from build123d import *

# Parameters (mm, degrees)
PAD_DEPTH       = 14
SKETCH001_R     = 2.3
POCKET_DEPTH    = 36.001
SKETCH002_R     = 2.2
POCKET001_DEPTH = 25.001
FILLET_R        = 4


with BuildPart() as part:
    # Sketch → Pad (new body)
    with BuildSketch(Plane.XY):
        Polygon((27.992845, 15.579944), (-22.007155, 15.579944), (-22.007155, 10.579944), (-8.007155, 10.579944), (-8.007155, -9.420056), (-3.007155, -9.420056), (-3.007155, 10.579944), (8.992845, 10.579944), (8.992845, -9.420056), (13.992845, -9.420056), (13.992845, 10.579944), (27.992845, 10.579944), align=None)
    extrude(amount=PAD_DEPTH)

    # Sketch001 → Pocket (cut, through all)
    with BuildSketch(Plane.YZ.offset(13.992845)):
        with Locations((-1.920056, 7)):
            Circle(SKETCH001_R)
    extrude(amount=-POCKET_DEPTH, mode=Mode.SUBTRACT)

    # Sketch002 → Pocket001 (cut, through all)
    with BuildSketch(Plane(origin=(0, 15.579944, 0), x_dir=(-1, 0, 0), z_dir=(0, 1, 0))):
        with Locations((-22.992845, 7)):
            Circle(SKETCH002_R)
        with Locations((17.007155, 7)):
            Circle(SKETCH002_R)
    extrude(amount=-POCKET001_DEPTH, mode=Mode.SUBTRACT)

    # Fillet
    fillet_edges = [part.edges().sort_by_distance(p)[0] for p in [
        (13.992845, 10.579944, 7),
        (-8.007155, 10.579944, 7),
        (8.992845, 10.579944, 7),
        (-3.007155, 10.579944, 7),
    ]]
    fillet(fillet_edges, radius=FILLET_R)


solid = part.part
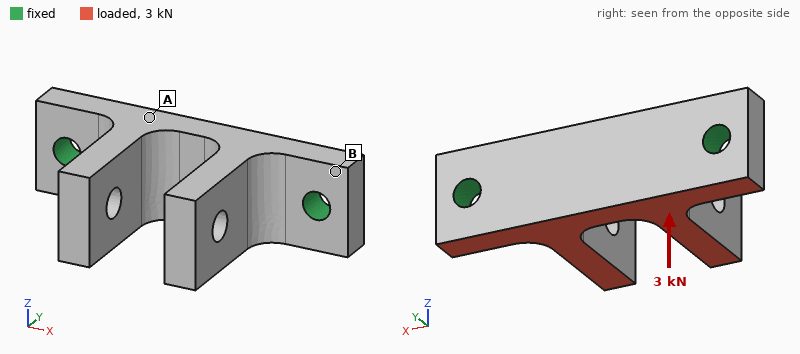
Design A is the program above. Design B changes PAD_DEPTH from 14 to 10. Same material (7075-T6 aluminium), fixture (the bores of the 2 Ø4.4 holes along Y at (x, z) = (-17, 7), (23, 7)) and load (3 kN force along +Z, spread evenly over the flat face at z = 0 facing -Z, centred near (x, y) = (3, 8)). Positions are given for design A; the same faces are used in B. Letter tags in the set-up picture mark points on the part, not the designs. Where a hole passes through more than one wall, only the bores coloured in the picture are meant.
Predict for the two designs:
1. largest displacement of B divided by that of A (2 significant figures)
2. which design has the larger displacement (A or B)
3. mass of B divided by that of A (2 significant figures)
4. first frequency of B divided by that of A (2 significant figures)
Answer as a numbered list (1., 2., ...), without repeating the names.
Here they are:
1. 1.8
2. B
3. 0.70
4. 0.93
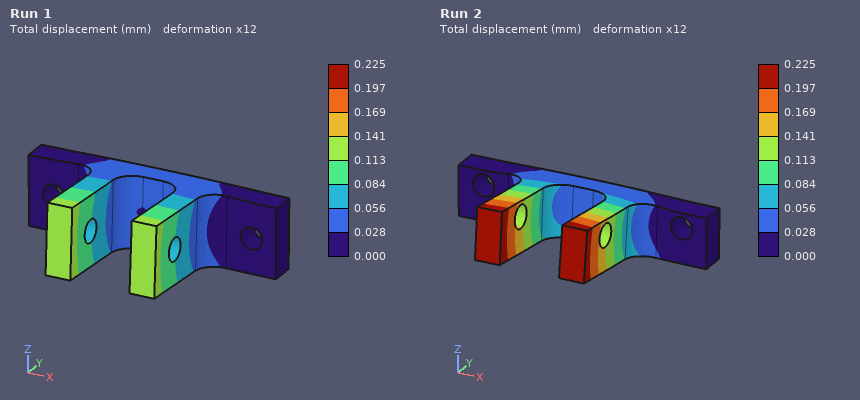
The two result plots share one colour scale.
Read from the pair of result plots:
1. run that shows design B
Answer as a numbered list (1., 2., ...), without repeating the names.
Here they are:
1. Run 2
